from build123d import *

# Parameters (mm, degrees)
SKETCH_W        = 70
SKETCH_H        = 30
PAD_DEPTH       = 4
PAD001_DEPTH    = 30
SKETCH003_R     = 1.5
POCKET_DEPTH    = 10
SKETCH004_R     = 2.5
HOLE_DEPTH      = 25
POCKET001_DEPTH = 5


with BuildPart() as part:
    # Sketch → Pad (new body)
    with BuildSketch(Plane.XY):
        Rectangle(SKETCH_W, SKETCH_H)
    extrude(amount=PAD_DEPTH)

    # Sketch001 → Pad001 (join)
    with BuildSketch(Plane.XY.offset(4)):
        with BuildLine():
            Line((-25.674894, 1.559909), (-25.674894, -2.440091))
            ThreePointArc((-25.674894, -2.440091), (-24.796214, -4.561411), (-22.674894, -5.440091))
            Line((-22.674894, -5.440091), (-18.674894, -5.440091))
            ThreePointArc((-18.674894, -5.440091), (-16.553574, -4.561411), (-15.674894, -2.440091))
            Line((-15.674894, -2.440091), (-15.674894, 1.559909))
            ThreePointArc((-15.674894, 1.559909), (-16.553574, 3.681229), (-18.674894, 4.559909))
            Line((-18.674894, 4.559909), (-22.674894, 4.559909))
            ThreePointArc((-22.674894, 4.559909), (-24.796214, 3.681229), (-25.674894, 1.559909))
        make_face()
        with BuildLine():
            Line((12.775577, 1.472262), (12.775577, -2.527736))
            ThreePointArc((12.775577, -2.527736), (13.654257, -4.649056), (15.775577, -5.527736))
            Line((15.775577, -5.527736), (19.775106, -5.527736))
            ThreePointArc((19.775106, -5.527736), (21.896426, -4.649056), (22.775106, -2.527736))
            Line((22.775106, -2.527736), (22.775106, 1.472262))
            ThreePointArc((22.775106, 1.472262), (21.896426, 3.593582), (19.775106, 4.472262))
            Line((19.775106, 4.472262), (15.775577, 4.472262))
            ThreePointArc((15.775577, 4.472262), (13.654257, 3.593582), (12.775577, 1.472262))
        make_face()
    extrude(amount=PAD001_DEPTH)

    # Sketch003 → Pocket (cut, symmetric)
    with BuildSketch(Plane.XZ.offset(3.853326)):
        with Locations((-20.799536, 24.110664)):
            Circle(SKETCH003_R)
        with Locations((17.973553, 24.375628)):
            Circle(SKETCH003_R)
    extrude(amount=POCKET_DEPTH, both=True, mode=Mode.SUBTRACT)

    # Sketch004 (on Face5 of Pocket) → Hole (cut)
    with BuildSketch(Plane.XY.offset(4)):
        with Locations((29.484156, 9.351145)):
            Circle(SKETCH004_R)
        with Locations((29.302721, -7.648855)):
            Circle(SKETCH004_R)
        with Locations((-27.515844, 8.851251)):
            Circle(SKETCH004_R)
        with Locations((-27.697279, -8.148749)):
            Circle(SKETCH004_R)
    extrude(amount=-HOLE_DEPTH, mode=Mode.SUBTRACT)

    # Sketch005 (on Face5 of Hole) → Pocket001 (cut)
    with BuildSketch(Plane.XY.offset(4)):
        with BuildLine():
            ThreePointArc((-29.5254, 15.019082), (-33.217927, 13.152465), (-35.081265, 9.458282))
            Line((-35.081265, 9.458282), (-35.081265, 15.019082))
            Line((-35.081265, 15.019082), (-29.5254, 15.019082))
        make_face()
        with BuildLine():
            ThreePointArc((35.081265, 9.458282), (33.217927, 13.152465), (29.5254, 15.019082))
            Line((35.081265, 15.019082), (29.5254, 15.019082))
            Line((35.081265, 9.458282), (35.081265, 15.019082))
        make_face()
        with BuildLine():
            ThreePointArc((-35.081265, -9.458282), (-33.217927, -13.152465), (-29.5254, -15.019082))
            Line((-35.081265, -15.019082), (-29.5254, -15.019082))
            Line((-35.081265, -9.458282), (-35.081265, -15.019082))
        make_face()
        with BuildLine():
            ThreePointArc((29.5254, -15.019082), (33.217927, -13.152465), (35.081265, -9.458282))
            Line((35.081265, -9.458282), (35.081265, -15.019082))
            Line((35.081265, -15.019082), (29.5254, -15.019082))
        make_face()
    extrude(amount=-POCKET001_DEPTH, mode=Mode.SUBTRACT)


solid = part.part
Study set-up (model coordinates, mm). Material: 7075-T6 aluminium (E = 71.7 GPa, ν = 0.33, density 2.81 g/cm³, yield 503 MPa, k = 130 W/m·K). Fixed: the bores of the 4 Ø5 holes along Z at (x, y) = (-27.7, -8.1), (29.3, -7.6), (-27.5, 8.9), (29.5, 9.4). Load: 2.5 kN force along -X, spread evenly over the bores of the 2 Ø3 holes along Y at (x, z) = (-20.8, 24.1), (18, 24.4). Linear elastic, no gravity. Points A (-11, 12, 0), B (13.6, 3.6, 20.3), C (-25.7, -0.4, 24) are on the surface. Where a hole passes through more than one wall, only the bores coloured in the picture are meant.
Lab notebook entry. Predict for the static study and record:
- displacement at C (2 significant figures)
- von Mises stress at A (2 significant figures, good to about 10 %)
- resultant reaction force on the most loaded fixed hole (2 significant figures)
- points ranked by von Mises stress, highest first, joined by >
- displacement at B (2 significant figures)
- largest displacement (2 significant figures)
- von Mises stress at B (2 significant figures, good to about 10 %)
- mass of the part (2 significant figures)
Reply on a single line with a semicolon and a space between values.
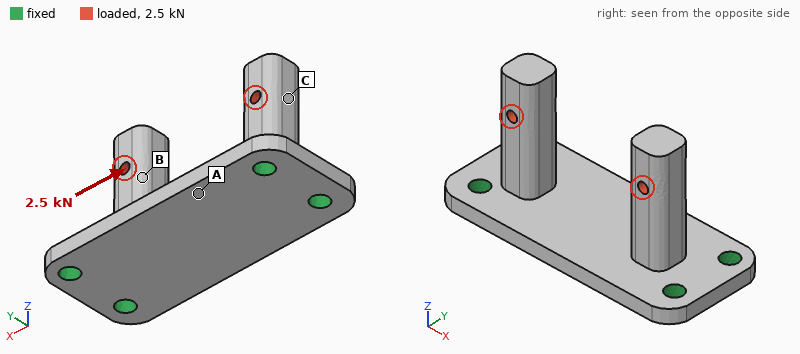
0.18 mm; 67 MPa; 920 N; A > B > C; 0.19 mm; 0.35 mm; 35 MPa; 38 g
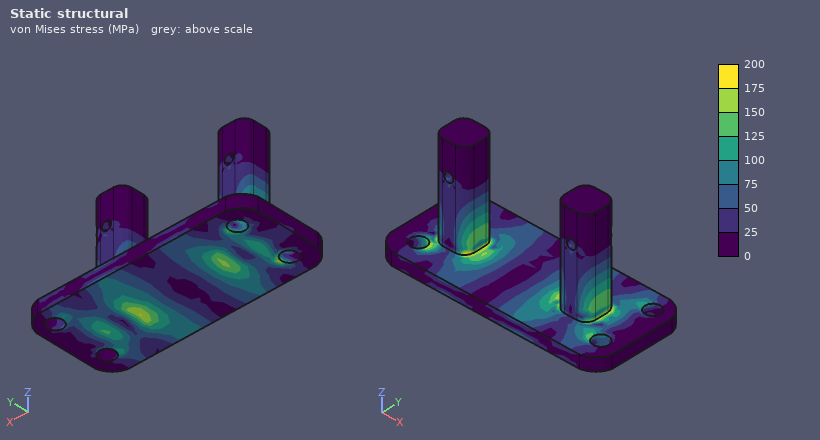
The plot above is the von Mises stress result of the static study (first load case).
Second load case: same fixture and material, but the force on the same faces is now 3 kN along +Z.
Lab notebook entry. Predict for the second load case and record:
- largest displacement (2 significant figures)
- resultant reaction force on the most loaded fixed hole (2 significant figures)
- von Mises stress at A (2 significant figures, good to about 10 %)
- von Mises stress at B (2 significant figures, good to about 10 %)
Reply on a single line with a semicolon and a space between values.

0.11 mm; 880 N; 16 MPa; 13 MPa
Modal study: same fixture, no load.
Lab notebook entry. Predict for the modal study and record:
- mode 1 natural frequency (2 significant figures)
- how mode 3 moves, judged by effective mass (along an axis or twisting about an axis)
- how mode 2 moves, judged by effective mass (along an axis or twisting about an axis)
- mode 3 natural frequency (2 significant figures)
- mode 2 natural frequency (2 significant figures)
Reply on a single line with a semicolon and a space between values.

3700 Hz; along X; along Y; 5200 Hz; 4900 Hz
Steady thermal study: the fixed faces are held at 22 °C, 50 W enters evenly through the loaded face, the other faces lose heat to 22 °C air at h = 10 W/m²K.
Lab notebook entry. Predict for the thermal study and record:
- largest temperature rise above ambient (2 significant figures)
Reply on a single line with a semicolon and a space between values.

64 K
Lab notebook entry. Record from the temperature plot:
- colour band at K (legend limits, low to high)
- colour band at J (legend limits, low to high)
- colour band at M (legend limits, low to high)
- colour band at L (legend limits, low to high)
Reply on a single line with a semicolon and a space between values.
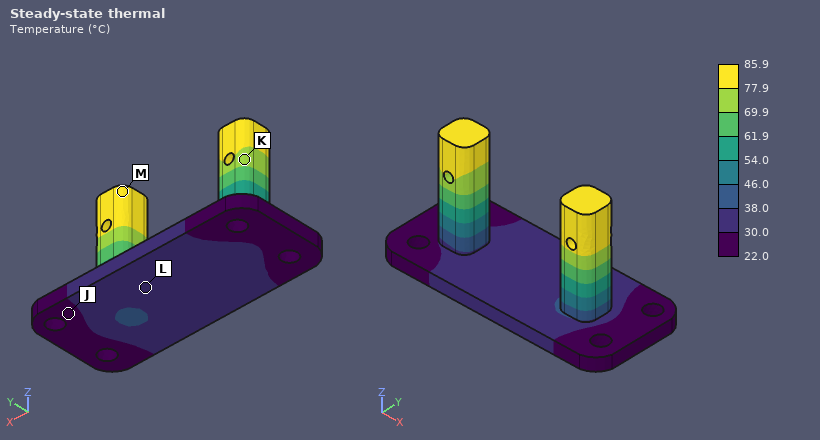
69.9 to 77.9 °C; 22.0 to 30.0 °C; 77.9 to 85.9 °C; 30.0 to 38.0 °C
